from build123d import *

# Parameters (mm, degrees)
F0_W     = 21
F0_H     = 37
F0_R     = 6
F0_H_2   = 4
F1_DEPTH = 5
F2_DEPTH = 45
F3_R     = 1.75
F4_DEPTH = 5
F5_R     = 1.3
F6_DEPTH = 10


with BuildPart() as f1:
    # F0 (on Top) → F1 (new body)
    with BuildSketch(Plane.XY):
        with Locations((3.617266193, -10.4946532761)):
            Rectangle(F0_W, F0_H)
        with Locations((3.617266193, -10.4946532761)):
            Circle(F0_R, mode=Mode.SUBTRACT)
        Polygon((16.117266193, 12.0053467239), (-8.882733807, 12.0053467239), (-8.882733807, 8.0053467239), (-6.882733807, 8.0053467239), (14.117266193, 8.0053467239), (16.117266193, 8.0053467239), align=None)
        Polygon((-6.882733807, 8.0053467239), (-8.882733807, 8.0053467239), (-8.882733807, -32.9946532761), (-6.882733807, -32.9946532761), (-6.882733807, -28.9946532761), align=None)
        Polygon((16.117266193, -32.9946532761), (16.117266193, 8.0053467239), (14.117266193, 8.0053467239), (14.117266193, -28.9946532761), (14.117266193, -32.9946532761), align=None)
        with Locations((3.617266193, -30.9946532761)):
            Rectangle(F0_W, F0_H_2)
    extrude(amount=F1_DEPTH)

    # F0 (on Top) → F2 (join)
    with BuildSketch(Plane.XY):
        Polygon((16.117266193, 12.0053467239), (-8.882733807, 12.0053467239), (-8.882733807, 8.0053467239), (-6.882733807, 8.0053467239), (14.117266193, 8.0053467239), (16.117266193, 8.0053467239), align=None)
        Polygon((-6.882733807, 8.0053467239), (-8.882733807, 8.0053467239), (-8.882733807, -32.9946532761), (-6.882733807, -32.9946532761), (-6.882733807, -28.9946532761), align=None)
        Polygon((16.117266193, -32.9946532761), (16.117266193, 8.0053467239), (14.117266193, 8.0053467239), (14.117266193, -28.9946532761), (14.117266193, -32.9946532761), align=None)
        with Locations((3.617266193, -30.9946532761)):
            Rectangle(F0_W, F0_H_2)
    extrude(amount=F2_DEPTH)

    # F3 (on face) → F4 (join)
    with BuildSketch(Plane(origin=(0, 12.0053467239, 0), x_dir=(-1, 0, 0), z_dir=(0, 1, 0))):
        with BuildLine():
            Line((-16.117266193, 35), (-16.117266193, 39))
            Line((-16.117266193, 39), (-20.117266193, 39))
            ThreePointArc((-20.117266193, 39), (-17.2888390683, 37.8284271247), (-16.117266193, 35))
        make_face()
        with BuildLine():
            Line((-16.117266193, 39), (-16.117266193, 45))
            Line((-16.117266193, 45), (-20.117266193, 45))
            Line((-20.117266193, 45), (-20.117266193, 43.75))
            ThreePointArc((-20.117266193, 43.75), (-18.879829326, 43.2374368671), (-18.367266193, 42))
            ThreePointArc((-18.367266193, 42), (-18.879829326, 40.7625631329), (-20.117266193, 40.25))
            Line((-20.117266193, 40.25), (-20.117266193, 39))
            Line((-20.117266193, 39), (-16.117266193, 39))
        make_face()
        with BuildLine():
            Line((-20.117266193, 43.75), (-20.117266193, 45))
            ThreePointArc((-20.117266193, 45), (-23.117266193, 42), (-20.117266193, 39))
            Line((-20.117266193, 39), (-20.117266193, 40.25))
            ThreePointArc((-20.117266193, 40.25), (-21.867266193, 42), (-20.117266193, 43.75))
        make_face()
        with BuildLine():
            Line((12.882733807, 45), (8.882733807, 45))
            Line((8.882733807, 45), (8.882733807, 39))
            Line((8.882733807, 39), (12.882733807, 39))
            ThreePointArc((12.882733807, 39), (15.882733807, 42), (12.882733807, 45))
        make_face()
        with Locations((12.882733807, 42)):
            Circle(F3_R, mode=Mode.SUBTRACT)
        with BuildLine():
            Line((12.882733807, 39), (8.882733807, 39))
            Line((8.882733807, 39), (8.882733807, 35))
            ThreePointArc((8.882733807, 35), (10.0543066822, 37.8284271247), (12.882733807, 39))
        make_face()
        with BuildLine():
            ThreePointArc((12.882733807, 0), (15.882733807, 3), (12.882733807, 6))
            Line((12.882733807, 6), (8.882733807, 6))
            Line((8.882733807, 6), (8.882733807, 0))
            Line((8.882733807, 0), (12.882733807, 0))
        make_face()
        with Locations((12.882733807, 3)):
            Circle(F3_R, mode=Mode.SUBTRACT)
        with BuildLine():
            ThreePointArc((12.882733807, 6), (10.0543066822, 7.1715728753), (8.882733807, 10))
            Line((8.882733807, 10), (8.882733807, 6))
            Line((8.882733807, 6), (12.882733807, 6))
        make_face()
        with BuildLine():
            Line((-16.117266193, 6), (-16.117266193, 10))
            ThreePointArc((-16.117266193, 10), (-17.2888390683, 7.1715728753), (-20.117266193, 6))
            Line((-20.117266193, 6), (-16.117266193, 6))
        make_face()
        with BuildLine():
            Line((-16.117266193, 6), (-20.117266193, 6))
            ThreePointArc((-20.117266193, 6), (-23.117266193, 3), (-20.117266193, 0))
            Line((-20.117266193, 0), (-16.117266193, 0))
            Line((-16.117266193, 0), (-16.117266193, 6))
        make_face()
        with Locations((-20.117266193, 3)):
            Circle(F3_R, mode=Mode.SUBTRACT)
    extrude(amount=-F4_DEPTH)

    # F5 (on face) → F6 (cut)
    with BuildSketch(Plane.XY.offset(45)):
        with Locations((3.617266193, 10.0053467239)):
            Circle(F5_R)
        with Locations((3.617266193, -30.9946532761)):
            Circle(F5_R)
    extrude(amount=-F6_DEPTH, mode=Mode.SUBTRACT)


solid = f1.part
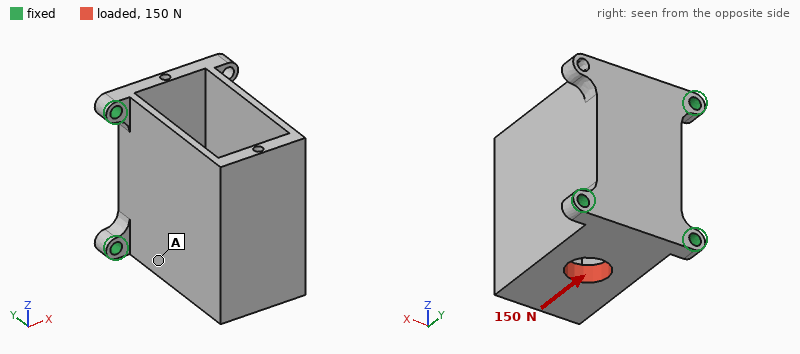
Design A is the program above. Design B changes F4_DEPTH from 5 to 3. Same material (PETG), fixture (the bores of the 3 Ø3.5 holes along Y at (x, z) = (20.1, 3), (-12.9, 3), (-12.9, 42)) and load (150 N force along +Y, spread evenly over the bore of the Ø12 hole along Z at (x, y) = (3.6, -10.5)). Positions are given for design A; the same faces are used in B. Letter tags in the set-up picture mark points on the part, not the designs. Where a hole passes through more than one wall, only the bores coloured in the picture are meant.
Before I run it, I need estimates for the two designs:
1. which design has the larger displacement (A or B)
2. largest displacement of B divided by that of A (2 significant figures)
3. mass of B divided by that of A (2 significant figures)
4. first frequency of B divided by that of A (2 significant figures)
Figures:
B
1.5
0.99
0.94
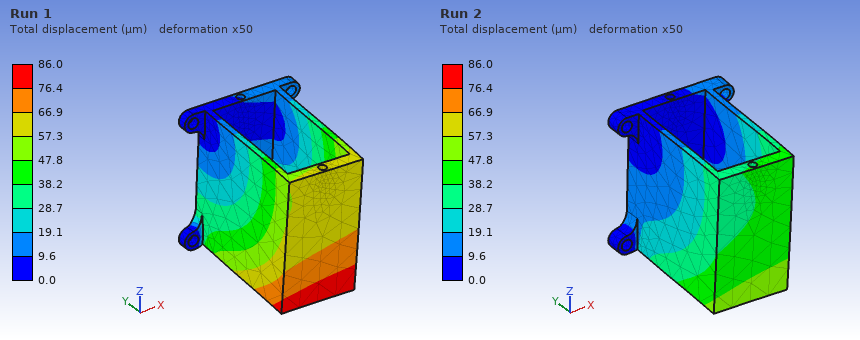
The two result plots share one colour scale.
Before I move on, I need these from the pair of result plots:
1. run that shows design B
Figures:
Run 1
